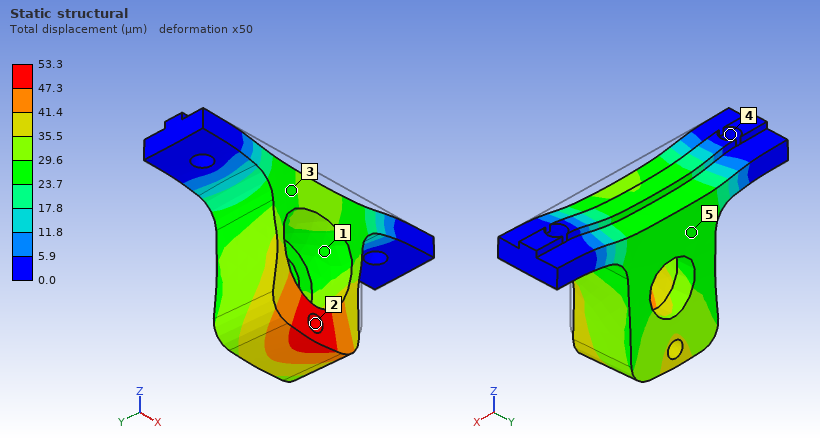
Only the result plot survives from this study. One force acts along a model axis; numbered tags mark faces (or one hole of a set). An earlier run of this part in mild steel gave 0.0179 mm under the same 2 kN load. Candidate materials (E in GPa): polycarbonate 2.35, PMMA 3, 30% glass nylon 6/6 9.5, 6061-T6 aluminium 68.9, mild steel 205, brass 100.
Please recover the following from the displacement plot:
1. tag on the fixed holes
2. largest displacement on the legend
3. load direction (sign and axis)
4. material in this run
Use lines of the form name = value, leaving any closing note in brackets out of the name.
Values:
tag on the fixed holes = 4
largest displacement on the legend = 53.3 µm
load direction = -Z
material in this run = 6061-T6 aluminium
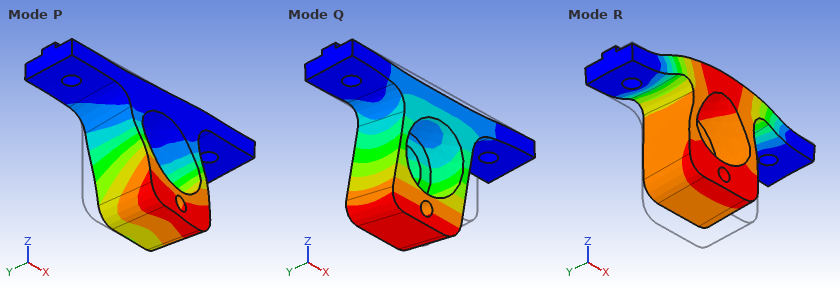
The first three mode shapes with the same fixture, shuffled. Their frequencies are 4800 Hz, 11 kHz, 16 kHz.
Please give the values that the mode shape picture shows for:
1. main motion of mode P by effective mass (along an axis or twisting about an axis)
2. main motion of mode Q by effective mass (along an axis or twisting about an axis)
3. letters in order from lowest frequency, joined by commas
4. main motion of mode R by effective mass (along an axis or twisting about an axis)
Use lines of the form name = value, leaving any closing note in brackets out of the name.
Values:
main motion of mode P by effective mass = along X
main motion of mode Q by effective mass = along Y
letters in order from lowest frequency, joined by commas = Q, P, R
main motion of mode R by effective mass = along Z
